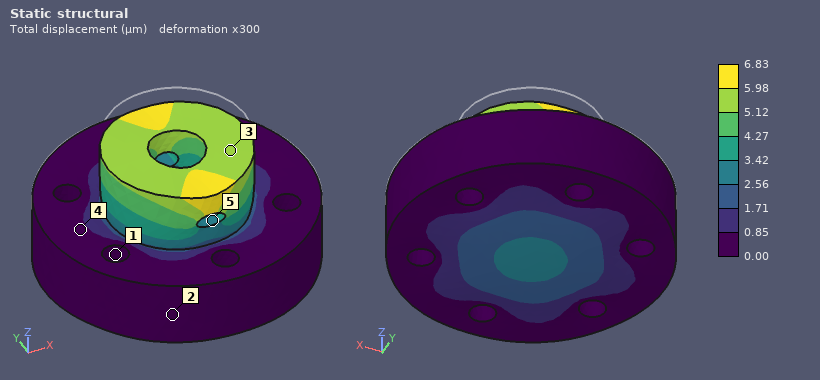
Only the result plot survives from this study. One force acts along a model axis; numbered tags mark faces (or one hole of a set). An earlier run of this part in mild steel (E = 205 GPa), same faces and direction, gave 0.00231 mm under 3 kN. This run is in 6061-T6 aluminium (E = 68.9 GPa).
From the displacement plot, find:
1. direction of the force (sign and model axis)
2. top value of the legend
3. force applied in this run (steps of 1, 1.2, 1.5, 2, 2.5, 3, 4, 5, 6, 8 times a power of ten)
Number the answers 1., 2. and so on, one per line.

1. -Z
2. 6.83 µm
3. 3 kN
